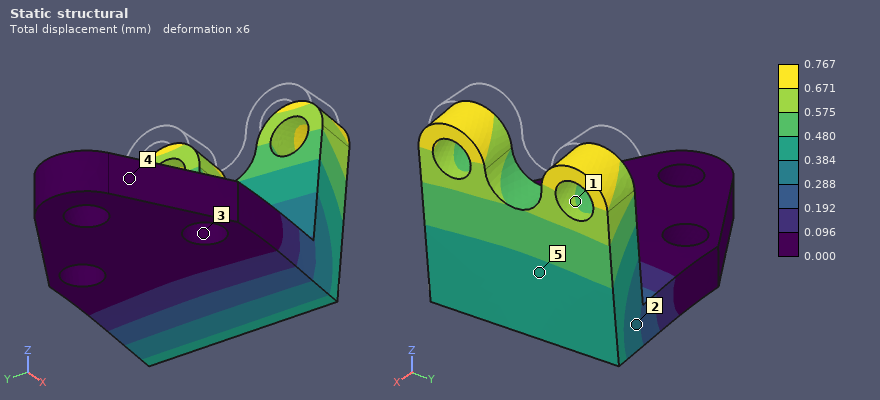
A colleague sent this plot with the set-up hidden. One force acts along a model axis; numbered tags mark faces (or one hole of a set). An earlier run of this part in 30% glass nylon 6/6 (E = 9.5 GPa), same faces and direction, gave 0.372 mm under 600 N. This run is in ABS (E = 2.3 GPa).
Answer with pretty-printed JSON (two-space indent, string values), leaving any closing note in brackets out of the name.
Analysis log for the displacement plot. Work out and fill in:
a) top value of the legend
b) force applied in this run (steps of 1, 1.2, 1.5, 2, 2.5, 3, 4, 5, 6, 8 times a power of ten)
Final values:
{
  "top value of the legend": "0.767 mm",
  "force applied in this run": "300 N"
}
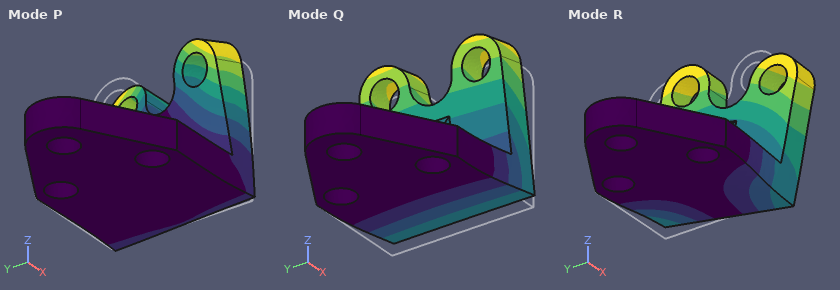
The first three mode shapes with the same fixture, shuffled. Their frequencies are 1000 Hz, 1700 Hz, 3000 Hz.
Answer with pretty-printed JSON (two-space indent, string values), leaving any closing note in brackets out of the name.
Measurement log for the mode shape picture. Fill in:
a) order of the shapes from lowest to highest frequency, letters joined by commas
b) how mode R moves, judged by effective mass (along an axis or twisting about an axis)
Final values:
{
  "order of the shapes from lowest to highest frequency, letters joined by commas": "Q, R, P",
  "how mode R moves, judged by effective mass": "along Y"
}
